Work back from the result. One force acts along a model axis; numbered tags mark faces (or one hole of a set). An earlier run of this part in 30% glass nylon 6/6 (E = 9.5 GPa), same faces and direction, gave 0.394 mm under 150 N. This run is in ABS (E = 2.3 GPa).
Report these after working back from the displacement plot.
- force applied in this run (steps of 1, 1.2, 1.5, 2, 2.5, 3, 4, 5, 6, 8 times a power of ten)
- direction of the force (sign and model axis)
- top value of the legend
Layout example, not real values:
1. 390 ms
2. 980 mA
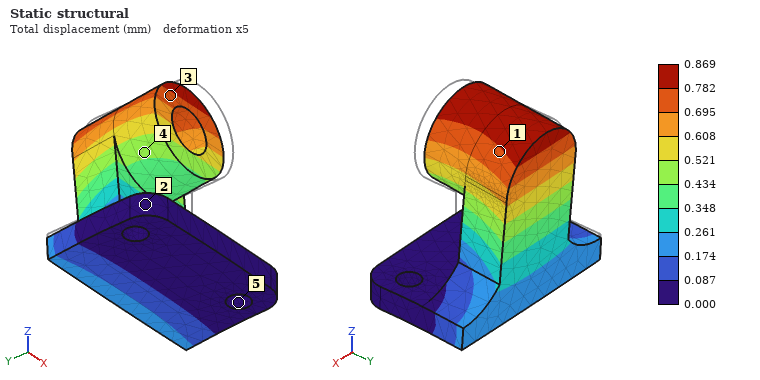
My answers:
1. 80 N
2. +Y
3. 0.869 mm
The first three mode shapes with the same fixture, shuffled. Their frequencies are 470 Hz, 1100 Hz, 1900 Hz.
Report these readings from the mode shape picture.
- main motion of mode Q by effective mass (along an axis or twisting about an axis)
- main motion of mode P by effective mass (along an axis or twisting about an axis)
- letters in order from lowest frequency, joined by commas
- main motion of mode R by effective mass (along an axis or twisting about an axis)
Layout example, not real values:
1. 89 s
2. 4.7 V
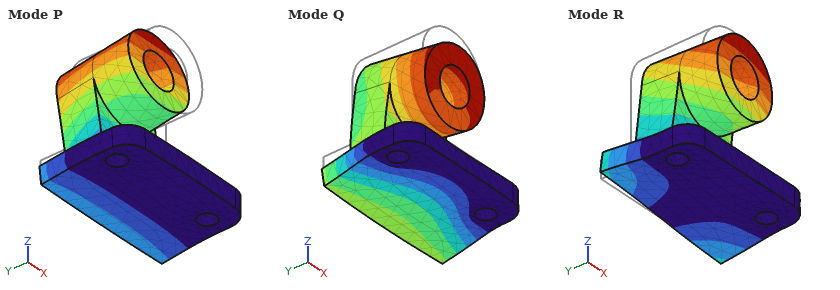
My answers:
1. along Z
2. along Y
3. P, R, Q
4. along X
